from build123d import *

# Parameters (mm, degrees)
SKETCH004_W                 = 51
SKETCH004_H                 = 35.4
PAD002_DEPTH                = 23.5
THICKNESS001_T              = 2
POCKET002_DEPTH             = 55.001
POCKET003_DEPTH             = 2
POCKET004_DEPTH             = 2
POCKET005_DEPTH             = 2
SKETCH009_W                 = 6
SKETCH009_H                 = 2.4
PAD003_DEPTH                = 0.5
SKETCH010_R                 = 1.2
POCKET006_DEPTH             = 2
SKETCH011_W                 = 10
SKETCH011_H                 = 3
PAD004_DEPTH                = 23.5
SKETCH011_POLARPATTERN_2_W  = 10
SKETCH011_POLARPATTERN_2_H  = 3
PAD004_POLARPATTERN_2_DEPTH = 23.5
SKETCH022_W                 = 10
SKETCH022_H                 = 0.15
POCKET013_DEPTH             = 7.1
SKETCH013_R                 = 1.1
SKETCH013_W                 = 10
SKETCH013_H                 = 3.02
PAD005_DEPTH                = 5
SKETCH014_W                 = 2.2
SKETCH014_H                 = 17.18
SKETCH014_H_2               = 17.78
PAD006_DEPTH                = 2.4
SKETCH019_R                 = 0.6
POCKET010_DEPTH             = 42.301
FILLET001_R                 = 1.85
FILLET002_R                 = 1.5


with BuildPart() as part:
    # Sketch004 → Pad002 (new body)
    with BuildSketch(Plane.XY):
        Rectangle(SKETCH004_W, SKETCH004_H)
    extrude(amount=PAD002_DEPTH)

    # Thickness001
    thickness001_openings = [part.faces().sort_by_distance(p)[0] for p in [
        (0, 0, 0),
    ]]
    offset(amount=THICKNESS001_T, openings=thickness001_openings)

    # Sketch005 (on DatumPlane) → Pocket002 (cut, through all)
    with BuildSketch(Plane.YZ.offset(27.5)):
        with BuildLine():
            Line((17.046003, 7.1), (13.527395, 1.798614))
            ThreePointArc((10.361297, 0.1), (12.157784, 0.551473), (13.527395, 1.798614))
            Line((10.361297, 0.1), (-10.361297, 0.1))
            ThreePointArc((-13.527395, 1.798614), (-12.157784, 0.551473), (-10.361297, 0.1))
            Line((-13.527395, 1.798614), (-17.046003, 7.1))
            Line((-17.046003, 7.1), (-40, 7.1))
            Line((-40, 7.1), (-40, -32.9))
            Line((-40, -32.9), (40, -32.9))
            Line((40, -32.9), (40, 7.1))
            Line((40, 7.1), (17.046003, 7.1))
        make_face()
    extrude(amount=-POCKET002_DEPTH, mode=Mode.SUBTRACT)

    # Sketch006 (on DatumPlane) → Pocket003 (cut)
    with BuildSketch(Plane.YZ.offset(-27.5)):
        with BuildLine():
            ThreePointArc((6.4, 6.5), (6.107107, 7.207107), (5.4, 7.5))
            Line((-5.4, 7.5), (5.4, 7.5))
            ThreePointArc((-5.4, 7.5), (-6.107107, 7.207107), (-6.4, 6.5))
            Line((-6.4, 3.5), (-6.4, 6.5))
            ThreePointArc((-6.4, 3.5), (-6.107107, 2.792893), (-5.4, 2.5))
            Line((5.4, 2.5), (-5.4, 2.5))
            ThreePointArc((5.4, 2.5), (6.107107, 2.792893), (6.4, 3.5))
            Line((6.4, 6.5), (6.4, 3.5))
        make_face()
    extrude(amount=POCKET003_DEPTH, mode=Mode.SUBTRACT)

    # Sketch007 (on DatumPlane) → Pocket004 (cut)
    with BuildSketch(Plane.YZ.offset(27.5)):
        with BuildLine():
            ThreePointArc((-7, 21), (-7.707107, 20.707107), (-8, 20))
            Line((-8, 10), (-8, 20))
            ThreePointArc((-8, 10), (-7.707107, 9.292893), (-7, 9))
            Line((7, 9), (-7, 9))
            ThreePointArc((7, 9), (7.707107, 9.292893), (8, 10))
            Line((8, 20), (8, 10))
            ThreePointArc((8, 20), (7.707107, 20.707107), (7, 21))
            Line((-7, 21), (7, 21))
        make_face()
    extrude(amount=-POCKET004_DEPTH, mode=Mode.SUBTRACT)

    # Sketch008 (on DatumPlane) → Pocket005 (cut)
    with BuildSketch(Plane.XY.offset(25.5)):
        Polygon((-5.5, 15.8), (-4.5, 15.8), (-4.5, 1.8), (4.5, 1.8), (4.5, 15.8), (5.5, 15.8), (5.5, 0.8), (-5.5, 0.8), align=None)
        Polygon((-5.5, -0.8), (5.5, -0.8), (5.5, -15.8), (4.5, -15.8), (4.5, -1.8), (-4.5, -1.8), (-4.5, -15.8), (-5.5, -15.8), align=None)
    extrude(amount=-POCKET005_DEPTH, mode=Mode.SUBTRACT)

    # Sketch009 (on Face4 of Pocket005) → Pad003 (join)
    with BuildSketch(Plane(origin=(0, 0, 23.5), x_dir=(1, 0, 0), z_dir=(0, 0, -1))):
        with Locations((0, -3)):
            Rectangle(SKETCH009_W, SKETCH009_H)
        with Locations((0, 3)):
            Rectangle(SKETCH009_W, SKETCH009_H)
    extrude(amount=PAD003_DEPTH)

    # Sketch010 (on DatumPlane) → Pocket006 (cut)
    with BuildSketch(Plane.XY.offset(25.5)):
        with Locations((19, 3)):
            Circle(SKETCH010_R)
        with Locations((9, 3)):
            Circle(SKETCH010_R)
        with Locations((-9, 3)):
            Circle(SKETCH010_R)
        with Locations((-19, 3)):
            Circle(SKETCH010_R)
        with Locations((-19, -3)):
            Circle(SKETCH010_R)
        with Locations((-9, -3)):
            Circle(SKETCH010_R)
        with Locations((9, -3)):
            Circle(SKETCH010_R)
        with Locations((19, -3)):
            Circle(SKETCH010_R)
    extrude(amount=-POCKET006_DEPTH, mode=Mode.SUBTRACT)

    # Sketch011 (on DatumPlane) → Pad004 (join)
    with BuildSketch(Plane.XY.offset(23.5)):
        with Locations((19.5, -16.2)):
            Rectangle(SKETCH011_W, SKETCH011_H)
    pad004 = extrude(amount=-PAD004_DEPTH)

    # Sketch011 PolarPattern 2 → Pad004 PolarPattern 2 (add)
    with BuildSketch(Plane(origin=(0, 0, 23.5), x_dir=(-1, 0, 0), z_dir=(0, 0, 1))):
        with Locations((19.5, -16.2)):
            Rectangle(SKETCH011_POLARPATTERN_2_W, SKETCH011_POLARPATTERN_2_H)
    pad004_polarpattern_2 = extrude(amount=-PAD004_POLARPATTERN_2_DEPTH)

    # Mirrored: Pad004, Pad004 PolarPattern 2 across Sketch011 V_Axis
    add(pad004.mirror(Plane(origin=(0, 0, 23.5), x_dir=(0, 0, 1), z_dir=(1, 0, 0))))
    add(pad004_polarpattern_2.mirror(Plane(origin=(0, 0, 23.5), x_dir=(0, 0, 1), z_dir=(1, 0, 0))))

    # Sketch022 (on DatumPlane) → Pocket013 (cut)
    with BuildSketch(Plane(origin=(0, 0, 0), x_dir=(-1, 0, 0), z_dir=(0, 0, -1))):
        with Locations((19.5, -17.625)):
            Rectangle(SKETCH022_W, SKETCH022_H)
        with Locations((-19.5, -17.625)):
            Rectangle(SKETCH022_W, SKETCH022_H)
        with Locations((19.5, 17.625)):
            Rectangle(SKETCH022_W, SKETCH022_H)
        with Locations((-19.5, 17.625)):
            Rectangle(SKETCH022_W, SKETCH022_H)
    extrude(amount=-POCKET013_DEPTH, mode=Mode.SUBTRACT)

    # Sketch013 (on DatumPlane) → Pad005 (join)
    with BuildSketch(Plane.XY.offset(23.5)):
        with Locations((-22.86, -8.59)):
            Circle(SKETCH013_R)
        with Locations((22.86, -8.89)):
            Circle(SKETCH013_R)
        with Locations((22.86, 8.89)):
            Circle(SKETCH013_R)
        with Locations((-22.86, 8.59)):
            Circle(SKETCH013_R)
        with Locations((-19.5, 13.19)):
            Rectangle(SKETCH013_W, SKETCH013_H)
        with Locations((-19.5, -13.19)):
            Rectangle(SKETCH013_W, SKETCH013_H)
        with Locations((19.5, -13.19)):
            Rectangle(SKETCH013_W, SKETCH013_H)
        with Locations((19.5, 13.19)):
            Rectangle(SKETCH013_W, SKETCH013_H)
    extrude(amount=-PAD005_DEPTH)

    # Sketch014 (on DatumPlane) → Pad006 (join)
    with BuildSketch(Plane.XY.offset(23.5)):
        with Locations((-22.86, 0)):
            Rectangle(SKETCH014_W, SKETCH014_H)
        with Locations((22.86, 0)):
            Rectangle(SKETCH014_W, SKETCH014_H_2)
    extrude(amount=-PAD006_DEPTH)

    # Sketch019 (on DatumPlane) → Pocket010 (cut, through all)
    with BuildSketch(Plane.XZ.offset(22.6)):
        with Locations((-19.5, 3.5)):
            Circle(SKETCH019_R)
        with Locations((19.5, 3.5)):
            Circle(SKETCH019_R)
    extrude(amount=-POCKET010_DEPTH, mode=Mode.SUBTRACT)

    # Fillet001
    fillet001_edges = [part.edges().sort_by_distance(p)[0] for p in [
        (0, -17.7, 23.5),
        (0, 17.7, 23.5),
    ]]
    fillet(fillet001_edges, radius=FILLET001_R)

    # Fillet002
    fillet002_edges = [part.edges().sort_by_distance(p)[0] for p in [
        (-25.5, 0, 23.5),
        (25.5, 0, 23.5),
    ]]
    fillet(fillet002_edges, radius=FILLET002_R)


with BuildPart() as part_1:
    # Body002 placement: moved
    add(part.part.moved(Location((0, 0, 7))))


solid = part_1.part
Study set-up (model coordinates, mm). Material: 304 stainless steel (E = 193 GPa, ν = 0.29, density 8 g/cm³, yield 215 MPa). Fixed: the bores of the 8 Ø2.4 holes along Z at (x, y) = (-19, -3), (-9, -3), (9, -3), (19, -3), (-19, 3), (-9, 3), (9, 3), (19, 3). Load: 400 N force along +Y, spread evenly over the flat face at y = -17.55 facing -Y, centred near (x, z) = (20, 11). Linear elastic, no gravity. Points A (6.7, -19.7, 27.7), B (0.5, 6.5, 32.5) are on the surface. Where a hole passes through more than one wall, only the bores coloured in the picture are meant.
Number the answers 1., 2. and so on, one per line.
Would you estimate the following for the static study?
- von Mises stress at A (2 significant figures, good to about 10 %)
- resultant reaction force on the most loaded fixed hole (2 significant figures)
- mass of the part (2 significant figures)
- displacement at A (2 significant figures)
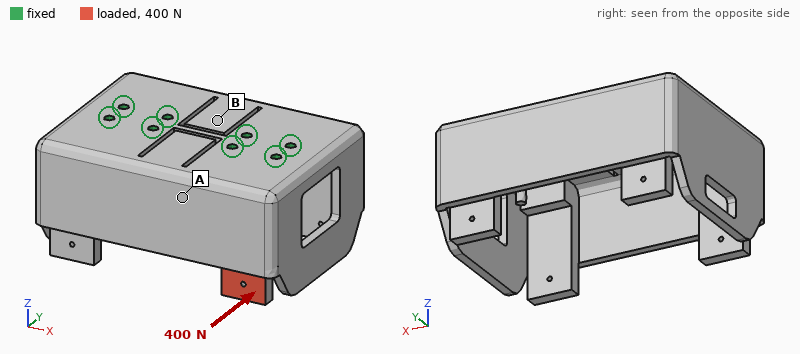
1. 36 MPa
2. 620 N
3. 110 g
4. 0.038 mm
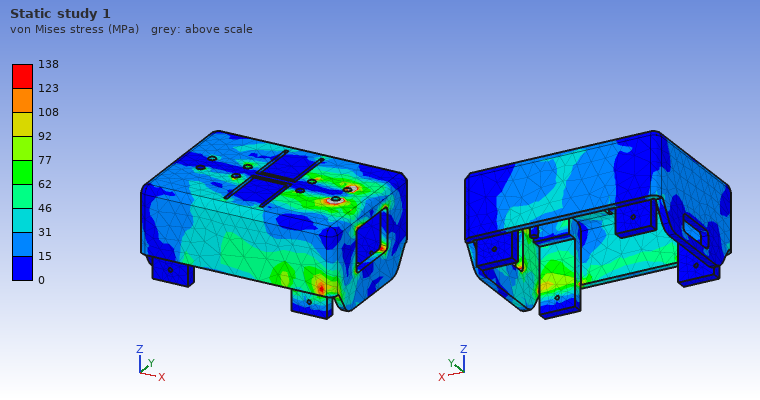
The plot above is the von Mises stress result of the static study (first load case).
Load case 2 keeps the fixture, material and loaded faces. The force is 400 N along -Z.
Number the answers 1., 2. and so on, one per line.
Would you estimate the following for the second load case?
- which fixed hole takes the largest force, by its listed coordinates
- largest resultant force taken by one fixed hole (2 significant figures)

1. (19, -3)
2. 620 N
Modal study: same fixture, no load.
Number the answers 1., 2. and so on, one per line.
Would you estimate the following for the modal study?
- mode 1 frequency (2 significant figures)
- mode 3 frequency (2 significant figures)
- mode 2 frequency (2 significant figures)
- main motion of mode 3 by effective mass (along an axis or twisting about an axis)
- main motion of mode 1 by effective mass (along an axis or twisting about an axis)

1. 2300 Hz
2. 4700 Hz
3. 2500 Hz
4. along X
5. along Y
